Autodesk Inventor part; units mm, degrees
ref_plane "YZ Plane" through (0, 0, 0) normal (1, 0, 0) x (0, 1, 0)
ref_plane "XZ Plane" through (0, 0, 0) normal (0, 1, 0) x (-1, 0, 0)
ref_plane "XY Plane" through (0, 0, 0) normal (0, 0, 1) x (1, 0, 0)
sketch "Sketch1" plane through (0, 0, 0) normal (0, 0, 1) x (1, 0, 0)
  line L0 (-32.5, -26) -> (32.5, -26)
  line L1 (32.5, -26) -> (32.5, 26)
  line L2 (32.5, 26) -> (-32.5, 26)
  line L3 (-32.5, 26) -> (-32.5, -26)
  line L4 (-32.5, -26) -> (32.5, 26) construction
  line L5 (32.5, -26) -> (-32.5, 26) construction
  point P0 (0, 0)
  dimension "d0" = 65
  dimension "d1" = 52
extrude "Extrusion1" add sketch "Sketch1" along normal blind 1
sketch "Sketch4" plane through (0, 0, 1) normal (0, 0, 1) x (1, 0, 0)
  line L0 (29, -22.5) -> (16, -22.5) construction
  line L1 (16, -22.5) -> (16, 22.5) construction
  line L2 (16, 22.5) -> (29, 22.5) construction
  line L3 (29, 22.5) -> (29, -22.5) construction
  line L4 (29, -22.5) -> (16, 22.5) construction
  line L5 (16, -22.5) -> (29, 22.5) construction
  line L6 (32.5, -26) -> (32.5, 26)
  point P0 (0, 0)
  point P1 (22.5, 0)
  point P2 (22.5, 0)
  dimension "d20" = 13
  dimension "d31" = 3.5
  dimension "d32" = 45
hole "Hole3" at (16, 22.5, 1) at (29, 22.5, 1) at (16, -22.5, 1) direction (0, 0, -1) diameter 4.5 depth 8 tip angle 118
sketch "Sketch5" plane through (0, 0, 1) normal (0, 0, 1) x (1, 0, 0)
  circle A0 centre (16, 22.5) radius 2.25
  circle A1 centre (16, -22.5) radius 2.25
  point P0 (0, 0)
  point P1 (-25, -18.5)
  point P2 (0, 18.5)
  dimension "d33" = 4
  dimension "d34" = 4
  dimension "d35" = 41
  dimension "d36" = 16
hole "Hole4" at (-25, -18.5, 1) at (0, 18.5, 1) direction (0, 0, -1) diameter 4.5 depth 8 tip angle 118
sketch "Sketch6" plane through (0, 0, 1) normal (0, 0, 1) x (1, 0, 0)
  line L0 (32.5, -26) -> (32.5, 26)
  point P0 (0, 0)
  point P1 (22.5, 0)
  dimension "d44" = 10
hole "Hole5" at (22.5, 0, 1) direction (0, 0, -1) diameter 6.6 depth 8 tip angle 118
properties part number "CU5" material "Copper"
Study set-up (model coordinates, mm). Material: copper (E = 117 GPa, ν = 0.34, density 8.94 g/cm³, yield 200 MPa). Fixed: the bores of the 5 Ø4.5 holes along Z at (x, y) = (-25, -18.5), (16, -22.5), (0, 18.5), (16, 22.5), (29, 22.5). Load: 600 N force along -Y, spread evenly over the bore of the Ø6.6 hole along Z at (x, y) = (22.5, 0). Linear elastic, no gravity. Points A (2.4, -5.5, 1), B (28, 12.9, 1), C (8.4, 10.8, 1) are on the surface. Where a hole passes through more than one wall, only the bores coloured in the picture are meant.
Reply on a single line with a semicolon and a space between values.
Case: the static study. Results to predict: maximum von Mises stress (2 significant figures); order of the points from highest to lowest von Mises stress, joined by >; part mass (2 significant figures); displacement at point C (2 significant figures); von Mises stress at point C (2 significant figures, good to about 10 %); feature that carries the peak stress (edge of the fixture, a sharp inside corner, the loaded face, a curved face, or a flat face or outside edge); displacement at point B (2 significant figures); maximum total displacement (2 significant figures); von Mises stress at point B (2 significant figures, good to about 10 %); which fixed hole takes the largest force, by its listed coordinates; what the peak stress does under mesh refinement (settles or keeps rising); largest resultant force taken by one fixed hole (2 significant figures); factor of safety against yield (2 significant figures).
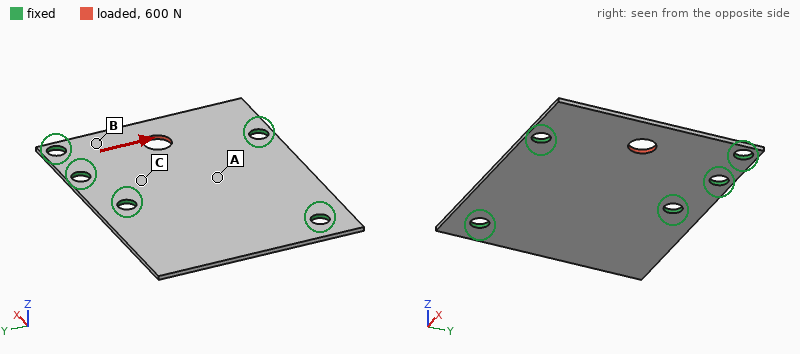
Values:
51 MPa; B > C > A; 29 g; 0.69 µm; 7.0 MPa; the loaded face; 1.3 µm; 4.2 µm; 19 MPa; (16, -22.5); settles; 220 N; 3.9
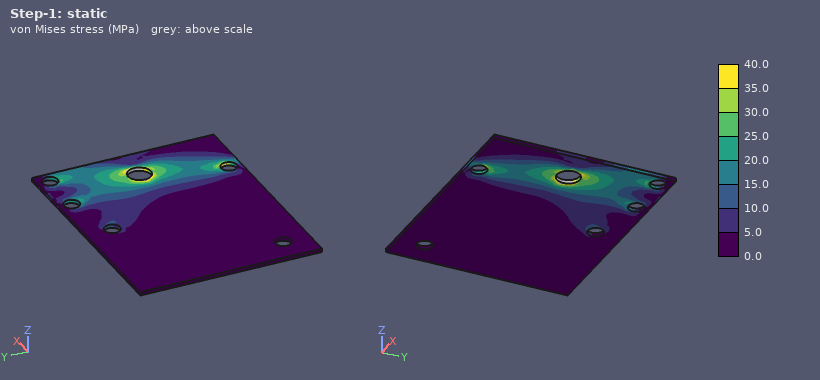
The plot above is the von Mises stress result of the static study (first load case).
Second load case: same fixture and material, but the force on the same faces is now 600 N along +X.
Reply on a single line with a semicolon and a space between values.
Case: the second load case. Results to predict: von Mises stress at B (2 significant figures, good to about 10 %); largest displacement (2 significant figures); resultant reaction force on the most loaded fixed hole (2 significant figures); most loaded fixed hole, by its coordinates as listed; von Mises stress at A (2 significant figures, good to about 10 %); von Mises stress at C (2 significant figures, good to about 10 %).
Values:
11 MPa; 6.8 µm; 190 N; (0, 18.5); 11 MPa; 17 MPa
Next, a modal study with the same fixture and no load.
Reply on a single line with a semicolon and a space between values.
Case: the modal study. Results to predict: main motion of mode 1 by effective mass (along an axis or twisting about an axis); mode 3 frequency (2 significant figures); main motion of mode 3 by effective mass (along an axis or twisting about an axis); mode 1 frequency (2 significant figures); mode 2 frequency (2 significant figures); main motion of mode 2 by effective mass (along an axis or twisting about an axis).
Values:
along Z; 2100 Hz; along Z; 910 Hz; 1900 Hz; along Z
